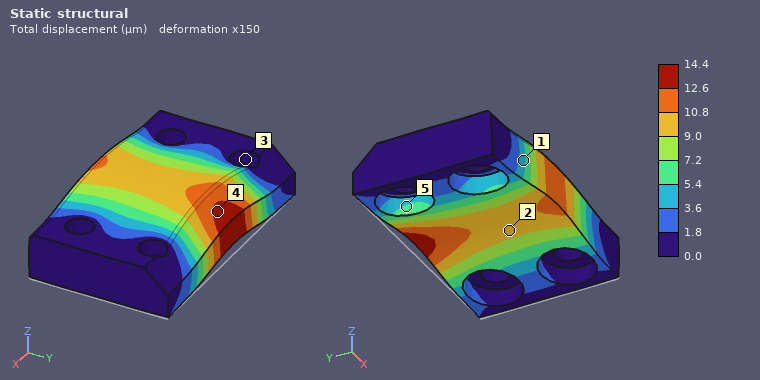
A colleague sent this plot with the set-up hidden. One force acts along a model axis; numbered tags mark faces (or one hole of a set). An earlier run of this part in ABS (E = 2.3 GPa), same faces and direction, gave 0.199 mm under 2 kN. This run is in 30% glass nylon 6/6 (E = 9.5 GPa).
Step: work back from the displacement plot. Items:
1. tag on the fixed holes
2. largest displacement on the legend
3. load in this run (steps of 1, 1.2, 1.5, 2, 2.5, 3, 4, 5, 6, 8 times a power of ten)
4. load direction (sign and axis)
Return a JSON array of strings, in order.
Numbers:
["3", "14.4 µm", "600 N", "+Z"]
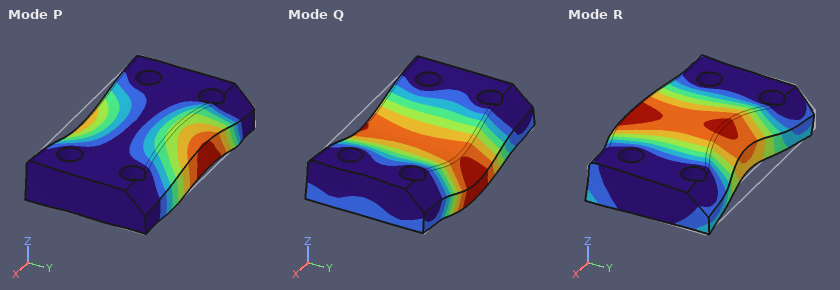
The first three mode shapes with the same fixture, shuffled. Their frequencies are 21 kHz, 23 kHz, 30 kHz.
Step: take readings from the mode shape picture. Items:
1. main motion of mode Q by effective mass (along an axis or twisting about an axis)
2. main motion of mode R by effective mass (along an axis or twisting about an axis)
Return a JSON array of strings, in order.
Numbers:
["along Z", "along Y"]
